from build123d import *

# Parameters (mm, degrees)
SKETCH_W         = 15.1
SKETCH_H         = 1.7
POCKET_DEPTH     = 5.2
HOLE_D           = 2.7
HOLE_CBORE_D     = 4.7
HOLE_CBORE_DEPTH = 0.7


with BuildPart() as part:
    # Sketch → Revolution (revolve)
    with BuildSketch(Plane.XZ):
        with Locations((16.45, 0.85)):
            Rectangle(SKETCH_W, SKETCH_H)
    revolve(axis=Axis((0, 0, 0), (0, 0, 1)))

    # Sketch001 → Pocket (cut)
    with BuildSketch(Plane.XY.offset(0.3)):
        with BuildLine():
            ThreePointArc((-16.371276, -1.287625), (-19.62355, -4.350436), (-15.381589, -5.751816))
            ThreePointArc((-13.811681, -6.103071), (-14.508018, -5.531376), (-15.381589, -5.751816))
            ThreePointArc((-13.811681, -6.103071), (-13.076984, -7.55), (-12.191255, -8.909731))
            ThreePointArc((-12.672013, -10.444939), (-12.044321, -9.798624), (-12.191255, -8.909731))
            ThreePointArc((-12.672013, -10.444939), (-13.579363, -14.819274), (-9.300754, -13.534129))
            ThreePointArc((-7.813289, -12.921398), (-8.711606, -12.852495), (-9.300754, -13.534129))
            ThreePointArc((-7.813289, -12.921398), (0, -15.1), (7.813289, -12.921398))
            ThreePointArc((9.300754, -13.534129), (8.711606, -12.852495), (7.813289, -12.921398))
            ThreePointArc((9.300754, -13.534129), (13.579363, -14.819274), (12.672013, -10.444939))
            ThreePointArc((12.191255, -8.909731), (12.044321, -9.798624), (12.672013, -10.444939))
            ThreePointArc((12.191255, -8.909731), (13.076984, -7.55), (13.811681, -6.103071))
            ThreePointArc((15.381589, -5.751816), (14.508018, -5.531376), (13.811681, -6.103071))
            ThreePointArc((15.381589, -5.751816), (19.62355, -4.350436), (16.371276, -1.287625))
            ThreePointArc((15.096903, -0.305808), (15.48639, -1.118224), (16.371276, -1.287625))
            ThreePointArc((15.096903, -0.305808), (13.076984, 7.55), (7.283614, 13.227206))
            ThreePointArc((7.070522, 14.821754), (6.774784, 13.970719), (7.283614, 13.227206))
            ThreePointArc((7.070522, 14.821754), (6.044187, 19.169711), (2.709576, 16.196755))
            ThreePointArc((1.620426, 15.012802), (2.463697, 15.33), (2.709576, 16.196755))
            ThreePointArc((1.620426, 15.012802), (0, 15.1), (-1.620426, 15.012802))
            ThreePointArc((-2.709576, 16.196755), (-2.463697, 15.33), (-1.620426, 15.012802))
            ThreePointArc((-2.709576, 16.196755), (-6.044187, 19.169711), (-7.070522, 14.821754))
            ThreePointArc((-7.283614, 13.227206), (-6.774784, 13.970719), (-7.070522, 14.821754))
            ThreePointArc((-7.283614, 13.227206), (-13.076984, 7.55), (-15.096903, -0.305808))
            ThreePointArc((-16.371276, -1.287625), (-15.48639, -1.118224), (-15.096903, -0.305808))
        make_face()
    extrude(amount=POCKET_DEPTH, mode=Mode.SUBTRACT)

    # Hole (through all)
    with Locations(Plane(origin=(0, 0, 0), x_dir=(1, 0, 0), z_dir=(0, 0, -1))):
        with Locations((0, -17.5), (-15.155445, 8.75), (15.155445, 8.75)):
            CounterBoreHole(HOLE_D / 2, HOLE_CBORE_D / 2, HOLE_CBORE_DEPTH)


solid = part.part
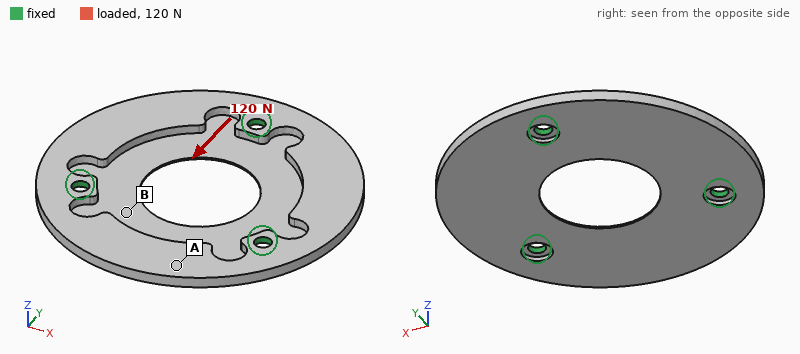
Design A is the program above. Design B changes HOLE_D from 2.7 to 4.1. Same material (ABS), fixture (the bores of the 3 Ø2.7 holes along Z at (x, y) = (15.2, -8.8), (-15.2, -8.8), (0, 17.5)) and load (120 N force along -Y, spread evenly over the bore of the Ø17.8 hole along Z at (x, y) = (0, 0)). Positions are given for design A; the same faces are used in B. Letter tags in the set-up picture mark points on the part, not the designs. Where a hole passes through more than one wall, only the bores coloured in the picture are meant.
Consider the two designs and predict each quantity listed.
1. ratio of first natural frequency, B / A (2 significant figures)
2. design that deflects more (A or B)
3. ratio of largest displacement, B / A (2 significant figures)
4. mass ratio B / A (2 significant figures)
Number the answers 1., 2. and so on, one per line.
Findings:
1. 1.1
2. A
3. 0.77
4. 0.99
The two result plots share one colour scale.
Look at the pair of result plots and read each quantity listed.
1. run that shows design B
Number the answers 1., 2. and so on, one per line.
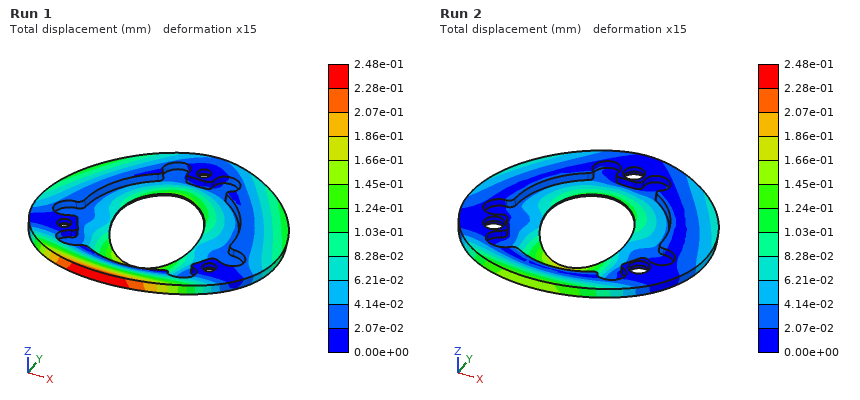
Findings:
1. Run 2
